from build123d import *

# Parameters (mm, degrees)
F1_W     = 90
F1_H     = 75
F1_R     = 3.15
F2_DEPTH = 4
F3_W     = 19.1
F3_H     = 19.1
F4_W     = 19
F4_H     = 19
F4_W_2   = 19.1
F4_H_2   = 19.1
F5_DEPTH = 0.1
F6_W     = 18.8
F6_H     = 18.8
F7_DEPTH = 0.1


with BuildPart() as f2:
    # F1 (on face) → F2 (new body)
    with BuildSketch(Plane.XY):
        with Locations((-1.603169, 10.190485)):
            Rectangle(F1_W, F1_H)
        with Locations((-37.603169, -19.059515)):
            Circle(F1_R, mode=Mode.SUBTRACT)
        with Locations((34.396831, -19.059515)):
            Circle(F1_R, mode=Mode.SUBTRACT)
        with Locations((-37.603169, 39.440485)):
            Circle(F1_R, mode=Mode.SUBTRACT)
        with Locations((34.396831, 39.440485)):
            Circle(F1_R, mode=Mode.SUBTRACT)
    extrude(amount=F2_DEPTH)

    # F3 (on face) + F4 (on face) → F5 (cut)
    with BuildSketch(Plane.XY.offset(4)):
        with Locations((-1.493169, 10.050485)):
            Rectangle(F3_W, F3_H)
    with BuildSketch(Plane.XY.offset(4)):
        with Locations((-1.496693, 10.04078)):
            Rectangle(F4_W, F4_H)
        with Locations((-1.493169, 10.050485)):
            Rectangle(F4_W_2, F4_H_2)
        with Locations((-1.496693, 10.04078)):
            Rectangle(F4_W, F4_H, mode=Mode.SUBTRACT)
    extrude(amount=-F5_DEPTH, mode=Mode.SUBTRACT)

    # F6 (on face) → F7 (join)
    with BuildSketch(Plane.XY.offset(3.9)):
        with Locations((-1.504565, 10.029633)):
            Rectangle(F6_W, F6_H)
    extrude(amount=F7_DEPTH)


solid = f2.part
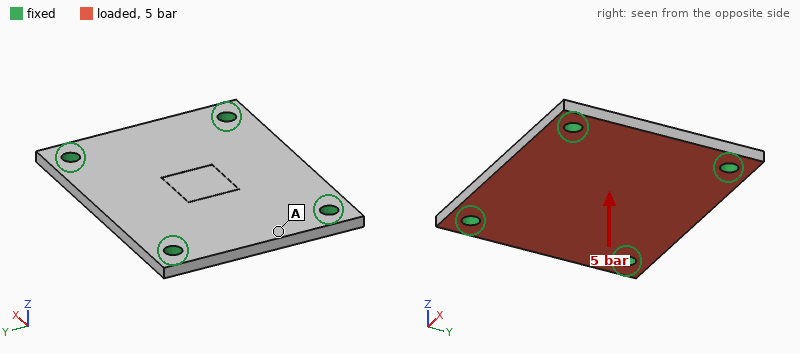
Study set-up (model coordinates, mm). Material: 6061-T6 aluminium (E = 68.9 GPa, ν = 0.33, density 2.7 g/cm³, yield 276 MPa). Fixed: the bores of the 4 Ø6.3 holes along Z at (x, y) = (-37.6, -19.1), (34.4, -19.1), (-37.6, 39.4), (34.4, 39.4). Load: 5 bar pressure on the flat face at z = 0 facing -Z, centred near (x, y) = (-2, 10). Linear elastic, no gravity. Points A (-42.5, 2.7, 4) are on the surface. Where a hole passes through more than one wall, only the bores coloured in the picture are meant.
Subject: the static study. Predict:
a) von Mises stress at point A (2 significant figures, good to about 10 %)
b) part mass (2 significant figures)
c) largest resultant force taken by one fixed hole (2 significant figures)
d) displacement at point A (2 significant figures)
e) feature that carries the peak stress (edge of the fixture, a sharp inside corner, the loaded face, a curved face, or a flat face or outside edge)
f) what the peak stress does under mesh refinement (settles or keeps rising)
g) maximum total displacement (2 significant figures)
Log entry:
22 MPa
72 g
830 N
0.031 mm
edge of the fixture
keeps rising
0.15 mm
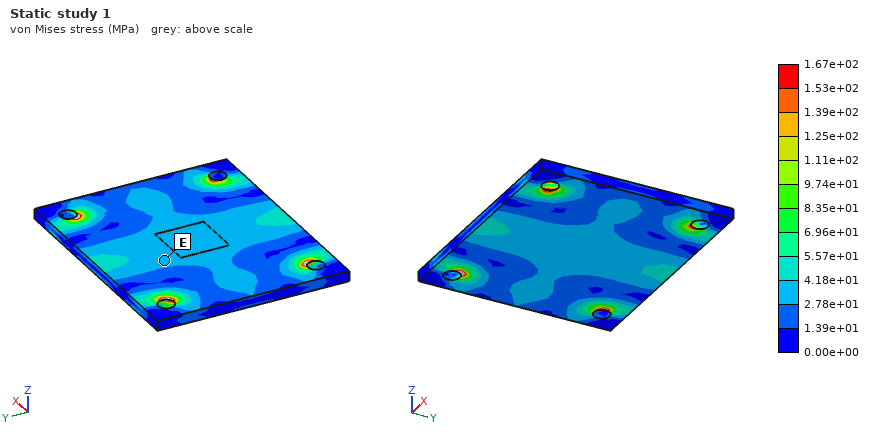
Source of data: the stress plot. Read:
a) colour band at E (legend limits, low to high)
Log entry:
2.78e+01 to 4.18e+01 MPa
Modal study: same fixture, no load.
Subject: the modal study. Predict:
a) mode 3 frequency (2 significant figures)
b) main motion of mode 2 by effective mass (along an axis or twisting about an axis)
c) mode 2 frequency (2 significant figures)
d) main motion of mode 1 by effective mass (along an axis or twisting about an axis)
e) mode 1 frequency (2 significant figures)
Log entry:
6200 Hz
twisting about X
5000 Hz
along Z
3400 Hz
